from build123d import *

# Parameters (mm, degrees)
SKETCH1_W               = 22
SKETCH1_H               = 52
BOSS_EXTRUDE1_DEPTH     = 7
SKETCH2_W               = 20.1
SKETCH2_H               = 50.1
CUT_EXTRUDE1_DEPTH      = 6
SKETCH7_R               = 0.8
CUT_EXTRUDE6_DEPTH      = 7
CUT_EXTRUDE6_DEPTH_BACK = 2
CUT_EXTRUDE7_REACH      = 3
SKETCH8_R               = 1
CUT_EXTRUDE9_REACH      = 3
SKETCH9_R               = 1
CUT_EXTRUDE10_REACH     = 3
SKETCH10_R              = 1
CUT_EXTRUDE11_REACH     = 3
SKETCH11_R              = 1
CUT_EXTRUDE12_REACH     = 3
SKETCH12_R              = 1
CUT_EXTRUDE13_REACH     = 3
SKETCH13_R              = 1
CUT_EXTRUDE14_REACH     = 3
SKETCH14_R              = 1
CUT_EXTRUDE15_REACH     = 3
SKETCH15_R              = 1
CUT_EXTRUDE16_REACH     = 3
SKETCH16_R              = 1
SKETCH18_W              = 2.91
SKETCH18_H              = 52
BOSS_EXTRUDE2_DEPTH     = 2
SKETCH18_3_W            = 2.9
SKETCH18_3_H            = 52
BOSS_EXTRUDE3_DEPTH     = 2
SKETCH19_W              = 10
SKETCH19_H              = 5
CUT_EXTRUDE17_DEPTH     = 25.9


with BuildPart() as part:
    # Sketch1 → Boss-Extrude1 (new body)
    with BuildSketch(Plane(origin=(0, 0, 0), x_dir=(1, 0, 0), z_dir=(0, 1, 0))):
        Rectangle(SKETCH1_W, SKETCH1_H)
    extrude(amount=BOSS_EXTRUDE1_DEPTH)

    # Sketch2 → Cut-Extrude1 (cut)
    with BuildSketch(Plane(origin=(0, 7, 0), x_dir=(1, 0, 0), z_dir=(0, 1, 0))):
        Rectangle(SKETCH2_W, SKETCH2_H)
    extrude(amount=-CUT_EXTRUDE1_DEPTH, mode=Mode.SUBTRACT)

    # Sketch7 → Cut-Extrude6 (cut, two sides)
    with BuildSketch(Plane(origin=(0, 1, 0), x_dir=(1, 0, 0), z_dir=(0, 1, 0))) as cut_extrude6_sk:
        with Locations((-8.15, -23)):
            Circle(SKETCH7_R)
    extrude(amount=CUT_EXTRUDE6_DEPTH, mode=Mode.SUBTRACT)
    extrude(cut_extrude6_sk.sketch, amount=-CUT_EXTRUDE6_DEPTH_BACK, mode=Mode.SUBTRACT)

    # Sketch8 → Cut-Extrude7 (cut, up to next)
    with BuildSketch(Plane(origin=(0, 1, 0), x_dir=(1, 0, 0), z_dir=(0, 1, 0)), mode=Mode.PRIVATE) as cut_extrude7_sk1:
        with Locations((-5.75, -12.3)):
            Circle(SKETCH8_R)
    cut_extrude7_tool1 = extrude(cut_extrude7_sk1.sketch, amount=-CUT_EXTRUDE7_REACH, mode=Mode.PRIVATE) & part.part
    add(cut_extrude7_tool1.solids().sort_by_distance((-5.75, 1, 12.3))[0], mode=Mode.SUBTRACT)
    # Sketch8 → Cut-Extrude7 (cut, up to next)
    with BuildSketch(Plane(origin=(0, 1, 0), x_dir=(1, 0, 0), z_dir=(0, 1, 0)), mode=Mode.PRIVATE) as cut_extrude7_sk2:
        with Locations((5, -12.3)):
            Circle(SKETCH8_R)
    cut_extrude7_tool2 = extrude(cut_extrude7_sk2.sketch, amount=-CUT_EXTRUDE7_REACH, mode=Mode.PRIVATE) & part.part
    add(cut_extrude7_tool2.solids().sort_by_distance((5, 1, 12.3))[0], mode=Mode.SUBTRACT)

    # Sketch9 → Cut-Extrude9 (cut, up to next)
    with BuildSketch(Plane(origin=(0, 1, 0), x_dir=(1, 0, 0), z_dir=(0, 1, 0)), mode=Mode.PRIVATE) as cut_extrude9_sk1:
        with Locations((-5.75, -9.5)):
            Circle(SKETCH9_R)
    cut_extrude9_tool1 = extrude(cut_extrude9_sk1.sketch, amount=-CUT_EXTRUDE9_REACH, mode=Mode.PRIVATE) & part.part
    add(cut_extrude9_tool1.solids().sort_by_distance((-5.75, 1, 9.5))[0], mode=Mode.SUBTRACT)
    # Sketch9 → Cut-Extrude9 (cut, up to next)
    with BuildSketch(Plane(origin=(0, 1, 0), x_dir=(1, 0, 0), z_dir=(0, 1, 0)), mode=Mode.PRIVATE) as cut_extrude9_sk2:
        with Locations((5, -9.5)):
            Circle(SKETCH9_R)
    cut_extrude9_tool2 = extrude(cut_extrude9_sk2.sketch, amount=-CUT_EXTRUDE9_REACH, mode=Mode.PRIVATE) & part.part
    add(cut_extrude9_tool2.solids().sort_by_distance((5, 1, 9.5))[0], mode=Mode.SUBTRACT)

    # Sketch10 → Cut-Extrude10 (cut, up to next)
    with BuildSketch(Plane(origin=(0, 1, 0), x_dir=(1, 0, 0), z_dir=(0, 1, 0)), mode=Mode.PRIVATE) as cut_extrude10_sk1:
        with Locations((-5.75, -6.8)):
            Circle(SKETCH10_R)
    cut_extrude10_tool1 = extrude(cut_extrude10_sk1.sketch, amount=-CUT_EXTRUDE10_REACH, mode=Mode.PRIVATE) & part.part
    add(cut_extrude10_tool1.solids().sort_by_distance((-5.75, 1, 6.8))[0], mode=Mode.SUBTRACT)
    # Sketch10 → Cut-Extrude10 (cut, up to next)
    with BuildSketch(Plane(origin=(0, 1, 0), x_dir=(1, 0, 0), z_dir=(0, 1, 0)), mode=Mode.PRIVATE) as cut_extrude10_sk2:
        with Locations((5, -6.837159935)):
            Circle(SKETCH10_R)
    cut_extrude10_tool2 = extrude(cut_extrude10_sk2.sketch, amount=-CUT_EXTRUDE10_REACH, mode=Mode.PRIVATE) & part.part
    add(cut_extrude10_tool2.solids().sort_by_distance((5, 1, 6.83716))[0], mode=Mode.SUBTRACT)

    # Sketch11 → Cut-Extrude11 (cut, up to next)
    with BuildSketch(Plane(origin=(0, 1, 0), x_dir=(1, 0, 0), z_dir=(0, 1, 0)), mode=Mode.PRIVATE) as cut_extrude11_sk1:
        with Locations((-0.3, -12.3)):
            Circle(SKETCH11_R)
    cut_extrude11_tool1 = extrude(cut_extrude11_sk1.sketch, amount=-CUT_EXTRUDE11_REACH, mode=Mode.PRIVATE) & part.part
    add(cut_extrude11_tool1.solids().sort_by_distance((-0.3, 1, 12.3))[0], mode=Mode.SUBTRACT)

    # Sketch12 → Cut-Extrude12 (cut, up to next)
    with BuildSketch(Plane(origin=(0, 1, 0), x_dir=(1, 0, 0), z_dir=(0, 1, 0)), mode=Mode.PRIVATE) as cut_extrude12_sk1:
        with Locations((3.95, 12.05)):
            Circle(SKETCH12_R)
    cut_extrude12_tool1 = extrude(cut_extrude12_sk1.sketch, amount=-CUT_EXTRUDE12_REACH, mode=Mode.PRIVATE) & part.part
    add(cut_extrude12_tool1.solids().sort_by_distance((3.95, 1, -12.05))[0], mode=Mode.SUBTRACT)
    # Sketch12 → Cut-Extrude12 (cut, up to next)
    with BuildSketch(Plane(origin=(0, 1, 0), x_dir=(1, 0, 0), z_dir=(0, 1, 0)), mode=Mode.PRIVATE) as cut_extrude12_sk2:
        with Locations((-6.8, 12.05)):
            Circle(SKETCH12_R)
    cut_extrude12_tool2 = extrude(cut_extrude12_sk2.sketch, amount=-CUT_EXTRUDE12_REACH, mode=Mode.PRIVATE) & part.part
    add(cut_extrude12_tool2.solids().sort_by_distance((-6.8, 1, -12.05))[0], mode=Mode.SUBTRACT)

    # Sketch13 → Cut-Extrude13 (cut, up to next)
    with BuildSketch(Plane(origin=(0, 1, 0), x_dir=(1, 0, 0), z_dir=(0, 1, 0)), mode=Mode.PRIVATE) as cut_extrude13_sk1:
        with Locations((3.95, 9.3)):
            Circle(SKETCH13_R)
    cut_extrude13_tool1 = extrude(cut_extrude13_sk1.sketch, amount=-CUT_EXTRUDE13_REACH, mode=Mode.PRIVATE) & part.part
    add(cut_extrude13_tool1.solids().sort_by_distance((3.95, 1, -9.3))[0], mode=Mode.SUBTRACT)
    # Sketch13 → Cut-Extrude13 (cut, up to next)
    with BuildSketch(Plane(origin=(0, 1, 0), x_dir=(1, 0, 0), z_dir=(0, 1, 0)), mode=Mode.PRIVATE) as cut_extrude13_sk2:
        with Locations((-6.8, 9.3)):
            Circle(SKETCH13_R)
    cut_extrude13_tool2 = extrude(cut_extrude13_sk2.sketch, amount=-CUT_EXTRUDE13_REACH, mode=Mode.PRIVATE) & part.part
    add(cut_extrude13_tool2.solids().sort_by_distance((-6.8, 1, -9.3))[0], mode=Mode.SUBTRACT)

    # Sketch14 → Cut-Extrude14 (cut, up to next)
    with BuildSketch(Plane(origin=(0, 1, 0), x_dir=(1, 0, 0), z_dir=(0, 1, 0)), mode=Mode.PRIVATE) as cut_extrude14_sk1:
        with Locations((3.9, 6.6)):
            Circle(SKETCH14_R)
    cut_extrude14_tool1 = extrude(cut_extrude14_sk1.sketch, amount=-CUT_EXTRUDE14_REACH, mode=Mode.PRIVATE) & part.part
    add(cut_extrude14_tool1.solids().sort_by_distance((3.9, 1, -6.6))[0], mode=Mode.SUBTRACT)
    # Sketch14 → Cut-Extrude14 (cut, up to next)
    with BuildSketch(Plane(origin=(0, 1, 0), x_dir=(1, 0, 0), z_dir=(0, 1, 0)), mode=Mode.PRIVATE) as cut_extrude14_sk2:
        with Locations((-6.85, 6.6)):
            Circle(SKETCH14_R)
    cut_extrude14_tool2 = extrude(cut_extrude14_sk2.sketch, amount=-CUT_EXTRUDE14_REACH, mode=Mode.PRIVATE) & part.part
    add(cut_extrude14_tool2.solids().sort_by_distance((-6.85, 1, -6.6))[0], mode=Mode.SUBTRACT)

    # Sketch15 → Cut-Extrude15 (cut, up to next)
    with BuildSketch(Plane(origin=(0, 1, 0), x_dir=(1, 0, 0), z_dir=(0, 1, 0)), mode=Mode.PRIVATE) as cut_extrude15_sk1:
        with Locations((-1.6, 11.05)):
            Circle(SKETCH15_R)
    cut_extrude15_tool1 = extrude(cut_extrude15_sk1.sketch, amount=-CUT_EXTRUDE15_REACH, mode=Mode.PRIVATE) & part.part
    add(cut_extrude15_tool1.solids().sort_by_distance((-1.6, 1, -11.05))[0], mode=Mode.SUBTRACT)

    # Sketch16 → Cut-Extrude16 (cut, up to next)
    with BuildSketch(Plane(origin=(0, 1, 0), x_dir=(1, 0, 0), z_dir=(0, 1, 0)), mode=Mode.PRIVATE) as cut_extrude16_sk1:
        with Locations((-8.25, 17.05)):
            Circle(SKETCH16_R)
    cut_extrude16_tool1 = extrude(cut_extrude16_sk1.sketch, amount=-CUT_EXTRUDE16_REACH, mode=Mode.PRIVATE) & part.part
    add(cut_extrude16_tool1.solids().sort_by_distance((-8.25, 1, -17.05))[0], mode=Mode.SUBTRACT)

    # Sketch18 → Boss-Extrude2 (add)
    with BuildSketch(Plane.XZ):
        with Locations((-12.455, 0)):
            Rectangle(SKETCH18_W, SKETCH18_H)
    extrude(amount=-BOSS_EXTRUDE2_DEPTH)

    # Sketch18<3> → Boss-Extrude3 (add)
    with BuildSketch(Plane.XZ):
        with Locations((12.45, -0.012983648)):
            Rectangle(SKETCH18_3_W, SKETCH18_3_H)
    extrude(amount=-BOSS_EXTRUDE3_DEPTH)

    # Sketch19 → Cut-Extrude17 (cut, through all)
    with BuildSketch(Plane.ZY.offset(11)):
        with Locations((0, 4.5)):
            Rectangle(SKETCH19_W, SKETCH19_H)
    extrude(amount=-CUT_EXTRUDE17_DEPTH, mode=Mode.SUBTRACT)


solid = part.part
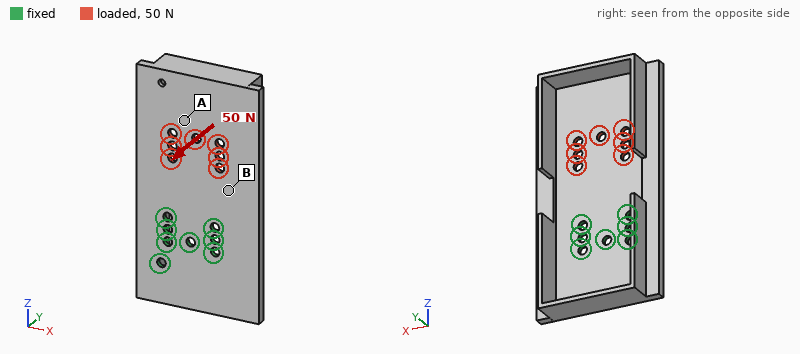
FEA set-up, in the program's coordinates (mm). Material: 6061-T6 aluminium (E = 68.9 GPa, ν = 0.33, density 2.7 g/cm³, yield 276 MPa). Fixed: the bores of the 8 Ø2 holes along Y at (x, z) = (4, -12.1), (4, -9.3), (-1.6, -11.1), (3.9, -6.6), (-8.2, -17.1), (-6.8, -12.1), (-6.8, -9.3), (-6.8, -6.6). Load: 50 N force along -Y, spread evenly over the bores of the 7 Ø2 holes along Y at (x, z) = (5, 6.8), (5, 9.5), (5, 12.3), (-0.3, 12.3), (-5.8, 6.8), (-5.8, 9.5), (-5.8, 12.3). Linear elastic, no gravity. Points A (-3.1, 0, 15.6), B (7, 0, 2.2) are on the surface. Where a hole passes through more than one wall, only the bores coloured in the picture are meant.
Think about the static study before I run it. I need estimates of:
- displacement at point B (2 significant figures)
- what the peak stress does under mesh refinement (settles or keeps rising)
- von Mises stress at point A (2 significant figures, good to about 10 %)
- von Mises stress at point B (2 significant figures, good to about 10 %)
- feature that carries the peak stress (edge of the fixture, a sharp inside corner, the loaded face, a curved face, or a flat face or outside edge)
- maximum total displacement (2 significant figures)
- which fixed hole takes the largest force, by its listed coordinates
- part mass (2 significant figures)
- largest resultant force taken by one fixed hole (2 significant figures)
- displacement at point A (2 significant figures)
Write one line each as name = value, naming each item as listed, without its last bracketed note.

displacement at point B = 0.076 mm
what the peak stress does under mesh refinement = keeps rising
von Mises stress at point A = 11 MPa
von Mises stress at point B = 29 MPa
feature that carries the peak stress = edge of the fixture
maximum total displacement = 0.39 mm
which fixed hole takes the largest force, by its listed coordinates = (-6.8, -6.6)
part mass = 6.6 g
largest resultant force taken by one fixed hole = 77 N
displacement at point A = 0.24 mm
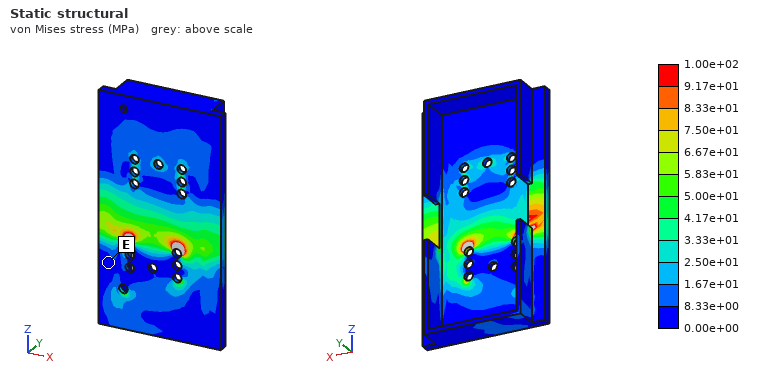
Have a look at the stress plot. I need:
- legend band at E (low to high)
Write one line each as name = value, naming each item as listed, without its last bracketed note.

legend band at E = 0.00e+00 to 8.33e+00 MPa
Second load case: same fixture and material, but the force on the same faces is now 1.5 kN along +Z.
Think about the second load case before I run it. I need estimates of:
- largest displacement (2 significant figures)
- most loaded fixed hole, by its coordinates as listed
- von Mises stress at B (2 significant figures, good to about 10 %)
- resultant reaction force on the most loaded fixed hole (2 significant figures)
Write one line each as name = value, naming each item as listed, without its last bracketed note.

largest displacement = 0.13 mm
most loaded fixed hole, by its coordinates as listed = (3.9, -6.6)
von Mises stress at B = 67 MPa
resultant reaction force on the most loaded fixed hole = 500 N
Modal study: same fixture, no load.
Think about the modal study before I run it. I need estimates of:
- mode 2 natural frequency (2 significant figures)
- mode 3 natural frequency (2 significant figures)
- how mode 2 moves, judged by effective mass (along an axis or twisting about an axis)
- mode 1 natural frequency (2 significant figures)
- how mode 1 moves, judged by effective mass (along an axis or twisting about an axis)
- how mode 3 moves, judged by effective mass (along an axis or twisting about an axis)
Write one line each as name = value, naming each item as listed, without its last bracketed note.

mode 2 natural frequency = 2100 Hz
mode 3 natural frequency = 4400 Hz
how mode 2 moves, judged by effective mass = twisting about Z
mode 1 natural frequency = 980 Hz
how mode 1 moves, judged by effective mass = along Y
how mode 3 moves, judged by effective mass = along Y
